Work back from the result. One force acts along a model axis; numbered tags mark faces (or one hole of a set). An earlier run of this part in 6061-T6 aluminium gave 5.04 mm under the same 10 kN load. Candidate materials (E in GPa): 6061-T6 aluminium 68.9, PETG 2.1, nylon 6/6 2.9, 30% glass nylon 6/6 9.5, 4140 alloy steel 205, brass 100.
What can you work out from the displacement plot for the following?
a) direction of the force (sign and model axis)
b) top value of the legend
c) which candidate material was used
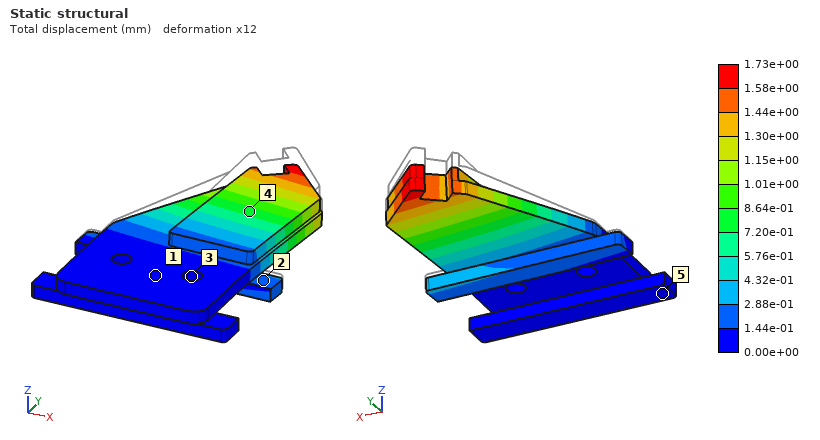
-Z
1.73e+00 mm
4140 alloy steel
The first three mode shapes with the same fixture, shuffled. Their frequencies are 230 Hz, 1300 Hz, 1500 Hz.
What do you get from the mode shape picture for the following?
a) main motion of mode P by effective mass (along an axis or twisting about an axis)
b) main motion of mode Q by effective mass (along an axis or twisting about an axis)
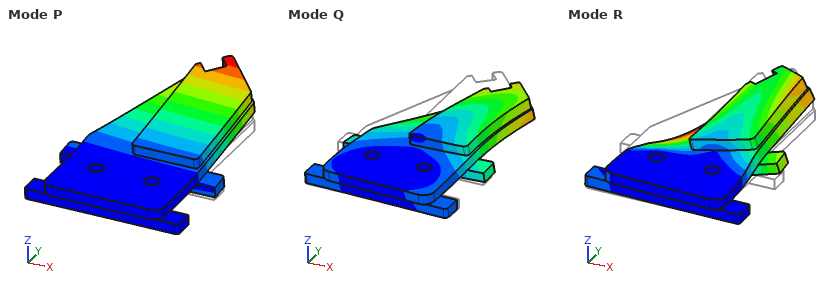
along Z
along X
